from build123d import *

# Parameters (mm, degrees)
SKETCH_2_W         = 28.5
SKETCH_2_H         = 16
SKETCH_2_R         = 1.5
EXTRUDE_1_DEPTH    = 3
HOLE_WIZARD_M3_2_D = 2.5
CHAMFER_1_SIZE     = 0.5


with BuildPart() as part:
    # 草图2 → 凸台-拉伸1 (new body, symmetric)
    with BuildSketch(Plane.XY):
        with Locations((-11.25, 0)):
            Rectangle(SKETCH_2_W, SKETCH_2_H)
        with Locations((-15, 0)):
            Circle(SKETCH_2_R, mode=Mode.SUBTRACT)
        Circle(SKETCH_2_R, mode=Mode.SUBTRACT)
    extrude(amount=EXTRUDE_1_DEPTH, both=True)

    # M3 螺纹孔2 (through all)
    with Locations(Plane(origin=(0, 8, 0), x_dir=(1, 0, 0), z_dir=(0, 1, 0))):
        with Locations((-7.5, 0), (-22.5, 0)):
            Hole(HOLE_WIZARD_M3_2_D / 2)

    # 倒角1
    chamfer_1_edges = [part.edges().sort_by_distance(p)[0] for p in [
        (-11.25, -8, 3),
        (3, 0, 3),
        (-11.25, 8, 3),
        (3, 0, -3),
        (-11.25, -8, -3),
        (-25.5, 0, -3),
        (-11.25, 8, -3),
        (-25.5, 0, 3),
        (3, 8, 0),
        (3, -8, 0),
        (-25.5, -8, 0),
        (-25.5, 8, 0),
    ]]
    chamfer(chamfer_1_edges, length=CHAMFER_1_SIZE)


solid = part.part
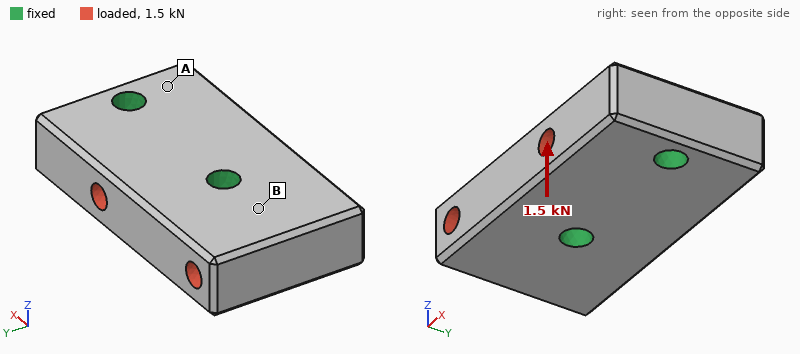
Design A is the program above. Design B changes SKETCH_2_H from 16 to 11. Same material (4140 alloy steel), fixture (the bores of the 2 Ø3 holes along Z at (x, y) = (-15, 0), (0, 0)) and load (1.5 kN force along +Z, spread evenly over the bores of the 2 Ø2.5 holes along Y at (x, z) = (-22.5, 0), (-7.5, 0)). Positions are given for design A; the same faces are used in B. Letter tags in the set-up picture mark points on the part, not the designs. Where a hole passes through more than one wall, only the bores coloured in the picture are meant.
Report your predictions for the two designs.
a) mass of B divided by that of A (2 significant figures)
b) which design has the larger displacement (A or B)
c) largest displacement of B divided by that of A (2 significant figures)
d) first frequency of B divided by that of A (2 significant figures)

0.67
B
1.2
1.1
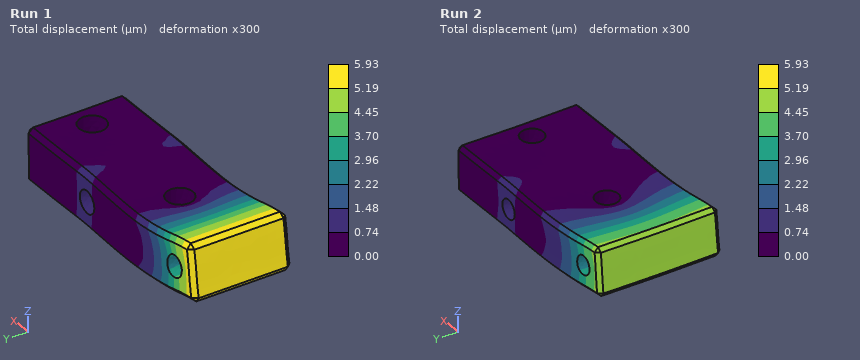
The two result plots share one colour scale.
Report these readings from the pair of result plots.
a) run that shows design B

Run 1
